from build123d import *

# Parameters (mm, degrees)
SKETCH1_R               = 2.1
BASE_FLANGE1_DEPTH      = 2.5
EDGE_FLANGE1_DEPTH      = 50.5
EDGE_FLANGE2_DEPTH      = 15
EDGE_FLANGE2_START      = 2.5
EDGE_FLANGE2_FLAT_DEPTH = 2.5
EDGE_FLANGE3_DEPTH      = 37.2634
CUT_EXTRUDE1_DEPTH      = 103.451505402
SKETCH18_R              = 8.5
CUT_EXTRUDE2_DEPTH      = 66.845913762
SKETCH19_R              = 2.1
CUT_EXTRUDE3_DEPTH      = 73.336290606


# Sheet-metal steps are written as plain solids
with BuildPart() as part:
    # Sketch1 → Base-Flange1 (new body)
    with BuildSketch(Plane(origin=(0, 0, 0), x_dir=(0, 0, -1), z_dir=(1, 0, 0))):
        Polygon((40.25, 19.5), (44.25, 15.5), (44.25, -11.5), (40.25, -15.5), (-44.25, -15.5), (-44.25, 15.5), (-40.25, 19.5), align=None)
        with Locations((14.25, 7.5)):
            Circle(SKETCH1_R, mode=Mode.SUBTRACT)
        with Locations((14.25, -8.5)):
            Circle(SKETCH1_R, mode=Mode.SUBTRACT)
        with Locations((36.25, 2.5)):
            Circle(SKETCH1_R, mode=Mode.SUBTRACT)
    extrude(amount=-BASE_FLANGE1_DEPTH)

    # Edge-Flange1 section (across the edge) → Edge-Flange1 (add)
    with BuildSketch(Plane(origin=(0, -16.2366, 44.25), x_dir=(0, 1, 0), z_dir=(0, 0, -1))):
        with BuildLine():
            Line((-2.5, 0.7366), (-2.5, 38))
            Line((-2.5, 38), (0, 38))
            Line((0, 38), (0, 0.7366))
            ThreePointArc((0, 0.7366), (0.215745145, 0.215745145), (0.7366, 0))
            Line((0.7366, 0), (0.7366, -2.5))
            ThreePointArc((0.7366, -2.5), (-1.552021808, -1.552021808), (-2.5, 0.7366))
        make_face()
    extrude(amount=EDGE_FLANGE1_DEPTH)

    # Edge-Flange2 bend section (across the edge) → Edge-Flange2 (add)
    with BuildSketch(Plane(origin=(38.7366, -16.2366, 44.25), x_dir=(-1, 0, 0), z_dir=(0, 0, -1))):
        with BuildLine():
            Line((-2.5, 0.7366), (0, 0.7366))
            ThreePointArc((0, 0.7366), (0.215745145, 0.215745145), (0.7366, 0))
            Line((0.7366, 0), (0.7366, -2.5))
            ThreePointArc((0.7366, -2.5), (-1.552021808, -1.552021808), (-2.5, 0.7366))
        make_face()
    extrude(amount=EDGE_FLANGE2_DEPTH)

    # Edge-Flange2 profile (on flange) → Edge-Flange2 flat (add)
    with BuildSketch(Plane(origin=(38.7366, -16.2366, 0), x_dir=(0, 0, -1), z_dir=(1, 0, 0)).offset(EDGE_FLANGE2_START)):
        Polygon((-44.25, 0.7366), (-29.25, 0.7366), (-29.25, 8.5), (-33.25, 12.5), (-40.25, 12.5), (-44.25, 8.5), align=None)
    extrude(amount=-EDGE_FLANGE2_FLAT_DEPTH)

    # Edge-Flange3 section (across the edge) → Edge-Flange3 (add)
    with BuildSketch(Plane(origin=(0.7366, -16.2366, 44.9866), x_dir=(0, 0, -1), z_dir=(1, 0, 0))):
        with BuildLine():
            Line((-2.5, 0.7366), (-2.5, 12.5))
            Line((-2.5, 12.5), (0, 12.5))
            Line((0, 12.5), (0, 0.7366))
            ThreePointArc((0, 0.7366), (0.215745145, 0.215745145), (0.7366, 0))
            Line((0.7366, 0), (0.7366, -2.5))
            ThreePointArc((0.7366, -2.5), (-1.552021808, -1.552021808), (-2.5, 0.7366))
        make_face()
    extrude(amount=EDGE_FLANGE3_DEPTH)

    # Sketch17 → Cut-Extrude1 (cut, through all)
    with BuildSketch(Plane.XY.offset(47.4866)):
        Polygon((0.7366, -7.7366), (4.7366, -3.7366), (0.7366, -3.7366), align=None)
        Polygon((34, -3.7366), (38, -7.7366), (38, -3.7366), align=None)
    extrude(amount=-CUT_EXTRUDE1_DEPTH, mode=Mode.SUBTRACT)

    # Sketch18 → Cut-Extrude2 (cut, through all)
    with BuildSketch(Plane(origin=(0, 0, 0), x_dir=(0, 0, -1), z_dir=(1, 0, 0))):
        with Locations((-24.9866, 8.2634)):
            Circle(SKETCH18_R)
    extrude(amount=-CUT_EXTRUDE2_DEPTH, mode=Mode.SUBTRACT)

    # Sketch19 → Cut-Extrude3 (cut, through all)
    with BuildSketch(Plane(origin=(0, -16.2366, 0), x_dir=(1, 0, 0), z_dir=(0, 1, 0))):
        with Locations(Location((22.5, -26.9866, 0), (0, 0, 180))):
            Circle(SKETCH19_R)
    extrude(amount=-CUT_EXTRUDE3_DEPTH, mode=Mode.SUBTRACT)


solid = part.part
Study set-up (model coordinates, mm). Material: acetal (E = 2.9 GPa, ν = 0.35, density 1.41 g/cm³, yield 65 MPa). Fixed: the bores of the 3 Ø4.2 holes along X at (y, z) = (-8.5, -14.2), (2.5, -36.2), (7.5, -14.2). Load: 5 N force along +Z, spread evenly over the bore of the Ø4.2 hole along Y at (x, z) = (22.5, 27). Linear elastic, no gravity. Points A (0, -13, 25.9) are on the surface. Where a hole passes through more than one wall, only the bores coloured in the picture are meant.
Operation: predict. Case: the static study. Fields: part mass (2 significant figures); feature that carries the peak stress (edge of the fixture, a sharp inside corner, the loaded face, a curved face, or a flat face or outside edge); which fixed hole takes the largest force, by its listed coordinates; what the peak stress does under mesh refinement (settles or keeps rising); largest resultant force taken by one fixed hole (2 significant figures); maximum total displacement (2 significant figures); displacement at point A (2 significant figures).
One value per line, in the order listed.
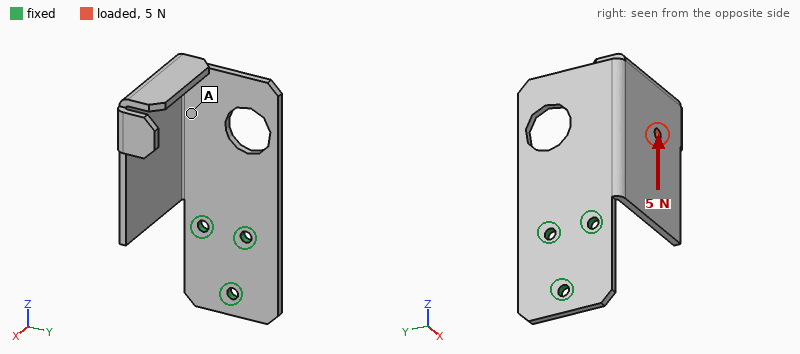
20 g
a sharp inside corner
(-8.5, -14.2)
keeps rising
6.2 N
1.2 mm
0.53 mm
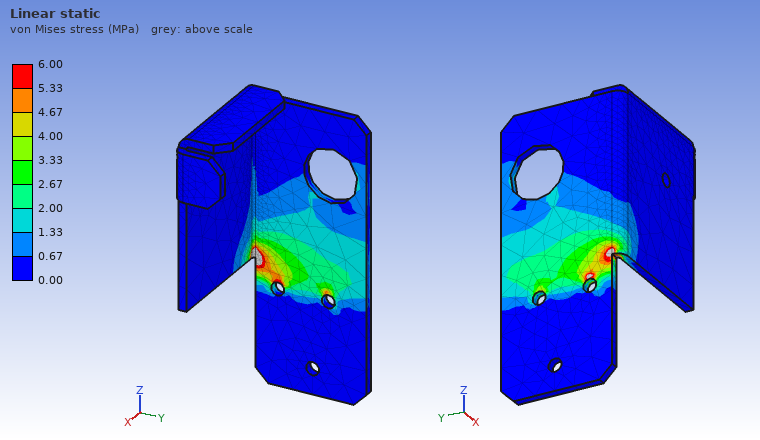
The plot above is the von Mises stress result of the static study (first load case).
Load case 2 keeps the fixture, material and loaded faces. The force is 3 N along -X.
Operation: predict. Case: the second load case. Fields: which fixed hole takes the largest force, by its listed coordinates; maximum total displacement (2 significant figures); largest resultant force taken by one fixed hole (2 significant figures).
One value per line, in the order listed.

(-8.5, -14.2)
1.0 mm
4.0 N
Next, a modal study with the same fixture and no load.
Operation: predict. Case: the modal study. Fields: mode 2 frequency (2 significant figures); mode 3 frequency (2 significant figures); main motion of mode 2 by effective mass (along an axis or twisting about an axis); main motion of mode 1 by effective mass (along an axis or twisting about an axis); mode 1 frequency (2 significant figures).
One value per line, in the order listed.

150 Hz
470 Hz
along Y
along X
88 Hz
